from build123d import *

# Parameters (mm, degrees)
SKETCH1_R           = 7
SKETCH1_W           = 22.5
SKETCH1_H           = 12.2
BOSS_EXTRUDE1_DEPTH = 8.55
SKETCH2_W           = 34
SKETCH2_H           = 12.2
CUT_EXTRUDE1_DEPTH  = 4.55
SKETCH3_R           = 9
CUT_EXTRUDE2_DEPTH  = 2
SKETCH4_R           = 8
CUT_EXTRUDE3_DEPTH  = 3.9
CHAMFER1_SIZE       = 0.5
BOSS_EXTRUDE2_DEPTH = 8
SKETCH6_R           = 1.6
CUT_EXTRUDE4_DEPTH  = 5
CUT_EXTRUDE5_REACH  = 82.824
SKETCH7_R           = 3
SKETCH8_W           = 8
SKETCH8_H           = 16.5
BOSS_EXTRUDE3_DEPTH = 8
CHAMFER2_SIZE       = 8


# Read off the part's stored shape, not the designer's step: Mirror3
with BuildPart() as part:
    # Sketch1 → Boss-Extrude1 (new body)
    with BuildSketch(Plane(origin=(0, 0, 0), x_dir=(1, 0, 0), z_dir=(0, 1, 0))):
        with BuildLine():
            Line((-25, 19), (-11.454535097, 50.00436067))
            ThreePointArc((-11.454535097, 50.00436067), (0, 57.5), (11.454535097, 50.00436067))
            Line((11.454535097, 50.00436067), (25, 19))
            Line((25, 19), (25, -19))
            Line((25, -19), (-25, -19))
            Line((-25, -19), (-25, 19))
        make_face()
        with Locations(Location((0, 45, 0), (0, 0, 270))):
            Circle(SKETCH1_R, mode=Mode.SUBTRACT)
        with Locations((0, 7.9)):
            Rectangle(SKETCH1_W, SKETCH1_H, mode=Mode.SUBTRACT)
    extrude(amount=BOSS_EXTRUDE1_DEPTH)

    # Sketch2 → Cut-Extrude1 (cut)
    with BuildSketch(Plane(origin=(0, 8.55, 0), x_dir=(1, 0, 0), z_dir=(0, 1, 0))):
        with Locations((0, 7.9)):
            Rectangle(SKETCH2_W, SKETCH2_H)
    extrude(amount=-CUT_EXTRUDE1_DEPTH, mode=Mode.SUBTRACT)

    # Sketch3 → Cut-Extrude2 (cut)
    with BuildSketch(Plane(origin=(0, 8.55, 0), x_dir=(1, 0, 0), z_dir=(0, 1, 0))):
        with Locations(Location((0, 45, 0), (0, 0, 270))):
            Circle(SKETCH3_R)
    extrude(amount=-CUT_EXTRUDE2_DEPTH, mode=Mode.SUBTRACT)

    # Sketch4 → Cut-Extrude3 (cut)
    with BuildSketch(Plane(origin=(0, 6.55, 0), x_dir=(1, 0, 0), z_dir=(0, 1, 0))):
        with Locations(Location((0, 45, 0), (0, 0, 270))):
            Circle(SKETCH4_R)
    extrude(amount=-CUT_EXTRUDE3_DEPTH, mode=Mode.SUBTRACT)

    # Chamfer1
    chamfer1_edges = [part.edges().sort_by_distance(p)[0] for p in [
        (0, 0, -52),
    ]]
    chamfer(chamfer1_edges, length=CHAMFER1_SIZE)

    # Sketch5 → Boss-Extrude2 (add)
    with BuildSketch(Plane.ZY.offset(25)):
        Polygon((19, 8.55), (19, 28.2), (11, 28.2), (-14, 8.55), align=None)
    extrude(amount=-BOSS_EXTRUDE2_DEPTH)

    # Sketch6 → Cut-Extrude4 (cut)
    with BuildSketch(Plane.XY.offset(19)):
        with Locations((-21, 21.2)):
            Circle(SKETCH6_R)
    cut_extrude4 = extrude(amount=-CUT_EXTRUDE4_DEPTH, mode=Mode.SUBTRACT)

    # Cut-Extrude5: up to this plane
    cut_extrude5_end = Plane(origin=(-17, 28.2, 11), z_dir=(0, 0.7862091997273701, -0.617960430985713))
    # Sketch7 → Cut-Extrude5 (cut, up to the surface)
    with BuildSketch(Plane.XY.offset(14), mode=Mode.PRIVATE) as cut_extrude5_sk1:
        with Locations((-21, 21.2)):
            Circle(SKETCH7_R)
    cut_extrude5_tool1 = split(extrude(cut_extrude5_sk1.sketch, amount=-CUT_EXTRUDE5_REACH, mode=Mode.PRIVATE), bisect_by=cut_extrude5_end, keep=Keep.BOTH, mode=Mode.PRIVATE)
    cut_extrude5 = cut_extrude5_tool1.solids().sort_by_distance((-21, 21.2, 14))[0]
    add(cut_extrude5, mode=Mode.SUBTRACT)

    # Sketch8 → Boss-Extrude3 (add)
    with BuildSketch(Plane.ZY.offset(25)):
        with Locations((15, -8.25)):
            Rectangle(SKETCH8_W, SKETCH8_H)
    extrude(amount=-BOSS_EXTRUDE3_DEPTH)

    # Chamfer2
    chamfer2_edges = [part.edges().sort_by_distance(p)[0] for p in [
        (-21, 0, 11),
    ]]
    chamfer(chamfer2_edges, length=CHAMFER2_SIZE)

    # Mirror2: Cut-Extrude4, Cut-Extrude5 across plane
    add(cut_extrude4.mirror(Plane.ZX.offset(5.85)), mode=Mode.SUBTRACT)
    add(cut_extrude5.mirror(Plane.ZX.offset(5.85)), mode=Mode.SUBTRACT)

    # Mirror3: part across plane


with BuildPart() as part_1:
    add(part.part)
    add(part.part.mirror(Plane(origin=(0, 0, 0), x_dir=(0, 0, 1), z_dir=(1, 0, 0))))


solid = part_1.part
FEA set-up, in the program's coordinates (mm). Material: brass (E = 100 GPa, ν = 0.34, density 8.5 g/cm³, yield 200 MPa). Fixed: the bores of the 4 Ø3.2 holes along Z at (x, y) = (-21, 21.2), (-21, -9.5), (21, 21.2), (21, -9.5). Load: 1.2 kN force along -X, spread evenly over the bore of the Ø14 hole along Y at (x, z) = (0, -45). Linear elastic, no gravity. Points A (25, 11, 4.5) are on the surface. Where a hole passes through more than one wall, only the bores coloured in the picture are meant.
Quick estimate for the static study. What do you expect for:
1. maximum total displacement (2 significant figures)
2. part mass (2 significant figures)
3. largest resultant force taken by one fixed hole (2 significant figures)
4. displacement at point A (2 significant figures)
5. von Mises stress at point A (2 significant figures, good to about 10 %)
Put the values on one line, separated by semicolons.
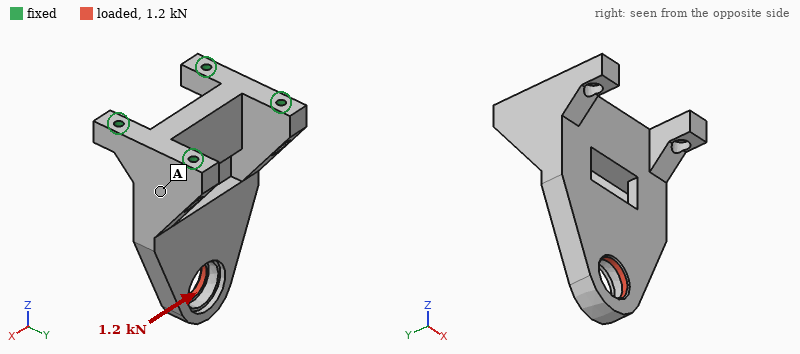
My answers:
43 µm; 260 g; 1.0 kN; 8.9 µm; 11 MPa
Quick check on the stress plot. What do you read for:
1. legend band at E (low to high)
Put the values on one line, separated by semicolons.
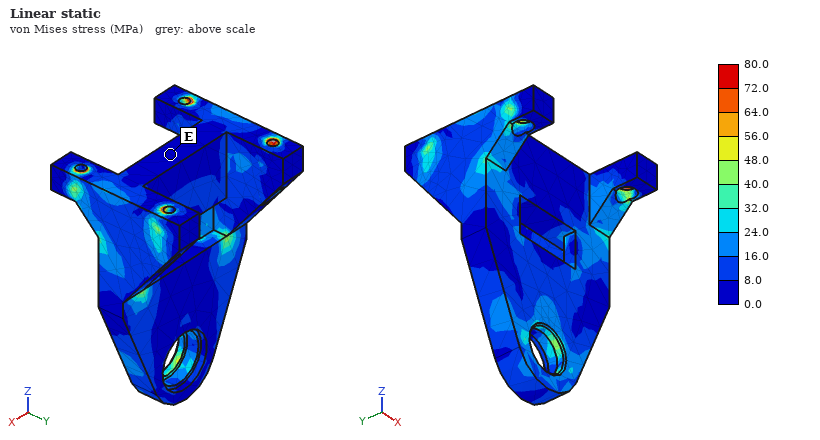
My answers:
0.0 to 8.0 MPa
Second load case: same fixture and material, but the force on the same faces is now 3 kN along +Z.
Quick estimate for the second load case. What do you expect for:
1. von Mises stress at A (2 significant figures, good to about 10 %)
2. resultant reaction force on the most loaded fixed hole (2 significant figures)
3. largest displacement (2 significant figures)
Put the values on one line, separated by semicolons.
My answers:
9.6 MPa; 1.1 kN; 0.10 mm
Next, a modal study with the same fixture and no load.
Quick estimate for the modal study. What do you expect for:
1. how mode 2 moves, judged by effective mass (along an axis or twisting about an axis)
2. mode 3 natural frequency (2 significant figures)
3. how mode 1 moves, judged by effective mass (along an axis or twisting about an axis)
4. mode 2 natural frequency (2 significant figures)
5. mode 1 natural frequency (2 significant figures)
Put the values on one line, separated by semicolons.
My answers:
along X; 5800 Hz; along Y; 3300 Hz; 1800 Hz
